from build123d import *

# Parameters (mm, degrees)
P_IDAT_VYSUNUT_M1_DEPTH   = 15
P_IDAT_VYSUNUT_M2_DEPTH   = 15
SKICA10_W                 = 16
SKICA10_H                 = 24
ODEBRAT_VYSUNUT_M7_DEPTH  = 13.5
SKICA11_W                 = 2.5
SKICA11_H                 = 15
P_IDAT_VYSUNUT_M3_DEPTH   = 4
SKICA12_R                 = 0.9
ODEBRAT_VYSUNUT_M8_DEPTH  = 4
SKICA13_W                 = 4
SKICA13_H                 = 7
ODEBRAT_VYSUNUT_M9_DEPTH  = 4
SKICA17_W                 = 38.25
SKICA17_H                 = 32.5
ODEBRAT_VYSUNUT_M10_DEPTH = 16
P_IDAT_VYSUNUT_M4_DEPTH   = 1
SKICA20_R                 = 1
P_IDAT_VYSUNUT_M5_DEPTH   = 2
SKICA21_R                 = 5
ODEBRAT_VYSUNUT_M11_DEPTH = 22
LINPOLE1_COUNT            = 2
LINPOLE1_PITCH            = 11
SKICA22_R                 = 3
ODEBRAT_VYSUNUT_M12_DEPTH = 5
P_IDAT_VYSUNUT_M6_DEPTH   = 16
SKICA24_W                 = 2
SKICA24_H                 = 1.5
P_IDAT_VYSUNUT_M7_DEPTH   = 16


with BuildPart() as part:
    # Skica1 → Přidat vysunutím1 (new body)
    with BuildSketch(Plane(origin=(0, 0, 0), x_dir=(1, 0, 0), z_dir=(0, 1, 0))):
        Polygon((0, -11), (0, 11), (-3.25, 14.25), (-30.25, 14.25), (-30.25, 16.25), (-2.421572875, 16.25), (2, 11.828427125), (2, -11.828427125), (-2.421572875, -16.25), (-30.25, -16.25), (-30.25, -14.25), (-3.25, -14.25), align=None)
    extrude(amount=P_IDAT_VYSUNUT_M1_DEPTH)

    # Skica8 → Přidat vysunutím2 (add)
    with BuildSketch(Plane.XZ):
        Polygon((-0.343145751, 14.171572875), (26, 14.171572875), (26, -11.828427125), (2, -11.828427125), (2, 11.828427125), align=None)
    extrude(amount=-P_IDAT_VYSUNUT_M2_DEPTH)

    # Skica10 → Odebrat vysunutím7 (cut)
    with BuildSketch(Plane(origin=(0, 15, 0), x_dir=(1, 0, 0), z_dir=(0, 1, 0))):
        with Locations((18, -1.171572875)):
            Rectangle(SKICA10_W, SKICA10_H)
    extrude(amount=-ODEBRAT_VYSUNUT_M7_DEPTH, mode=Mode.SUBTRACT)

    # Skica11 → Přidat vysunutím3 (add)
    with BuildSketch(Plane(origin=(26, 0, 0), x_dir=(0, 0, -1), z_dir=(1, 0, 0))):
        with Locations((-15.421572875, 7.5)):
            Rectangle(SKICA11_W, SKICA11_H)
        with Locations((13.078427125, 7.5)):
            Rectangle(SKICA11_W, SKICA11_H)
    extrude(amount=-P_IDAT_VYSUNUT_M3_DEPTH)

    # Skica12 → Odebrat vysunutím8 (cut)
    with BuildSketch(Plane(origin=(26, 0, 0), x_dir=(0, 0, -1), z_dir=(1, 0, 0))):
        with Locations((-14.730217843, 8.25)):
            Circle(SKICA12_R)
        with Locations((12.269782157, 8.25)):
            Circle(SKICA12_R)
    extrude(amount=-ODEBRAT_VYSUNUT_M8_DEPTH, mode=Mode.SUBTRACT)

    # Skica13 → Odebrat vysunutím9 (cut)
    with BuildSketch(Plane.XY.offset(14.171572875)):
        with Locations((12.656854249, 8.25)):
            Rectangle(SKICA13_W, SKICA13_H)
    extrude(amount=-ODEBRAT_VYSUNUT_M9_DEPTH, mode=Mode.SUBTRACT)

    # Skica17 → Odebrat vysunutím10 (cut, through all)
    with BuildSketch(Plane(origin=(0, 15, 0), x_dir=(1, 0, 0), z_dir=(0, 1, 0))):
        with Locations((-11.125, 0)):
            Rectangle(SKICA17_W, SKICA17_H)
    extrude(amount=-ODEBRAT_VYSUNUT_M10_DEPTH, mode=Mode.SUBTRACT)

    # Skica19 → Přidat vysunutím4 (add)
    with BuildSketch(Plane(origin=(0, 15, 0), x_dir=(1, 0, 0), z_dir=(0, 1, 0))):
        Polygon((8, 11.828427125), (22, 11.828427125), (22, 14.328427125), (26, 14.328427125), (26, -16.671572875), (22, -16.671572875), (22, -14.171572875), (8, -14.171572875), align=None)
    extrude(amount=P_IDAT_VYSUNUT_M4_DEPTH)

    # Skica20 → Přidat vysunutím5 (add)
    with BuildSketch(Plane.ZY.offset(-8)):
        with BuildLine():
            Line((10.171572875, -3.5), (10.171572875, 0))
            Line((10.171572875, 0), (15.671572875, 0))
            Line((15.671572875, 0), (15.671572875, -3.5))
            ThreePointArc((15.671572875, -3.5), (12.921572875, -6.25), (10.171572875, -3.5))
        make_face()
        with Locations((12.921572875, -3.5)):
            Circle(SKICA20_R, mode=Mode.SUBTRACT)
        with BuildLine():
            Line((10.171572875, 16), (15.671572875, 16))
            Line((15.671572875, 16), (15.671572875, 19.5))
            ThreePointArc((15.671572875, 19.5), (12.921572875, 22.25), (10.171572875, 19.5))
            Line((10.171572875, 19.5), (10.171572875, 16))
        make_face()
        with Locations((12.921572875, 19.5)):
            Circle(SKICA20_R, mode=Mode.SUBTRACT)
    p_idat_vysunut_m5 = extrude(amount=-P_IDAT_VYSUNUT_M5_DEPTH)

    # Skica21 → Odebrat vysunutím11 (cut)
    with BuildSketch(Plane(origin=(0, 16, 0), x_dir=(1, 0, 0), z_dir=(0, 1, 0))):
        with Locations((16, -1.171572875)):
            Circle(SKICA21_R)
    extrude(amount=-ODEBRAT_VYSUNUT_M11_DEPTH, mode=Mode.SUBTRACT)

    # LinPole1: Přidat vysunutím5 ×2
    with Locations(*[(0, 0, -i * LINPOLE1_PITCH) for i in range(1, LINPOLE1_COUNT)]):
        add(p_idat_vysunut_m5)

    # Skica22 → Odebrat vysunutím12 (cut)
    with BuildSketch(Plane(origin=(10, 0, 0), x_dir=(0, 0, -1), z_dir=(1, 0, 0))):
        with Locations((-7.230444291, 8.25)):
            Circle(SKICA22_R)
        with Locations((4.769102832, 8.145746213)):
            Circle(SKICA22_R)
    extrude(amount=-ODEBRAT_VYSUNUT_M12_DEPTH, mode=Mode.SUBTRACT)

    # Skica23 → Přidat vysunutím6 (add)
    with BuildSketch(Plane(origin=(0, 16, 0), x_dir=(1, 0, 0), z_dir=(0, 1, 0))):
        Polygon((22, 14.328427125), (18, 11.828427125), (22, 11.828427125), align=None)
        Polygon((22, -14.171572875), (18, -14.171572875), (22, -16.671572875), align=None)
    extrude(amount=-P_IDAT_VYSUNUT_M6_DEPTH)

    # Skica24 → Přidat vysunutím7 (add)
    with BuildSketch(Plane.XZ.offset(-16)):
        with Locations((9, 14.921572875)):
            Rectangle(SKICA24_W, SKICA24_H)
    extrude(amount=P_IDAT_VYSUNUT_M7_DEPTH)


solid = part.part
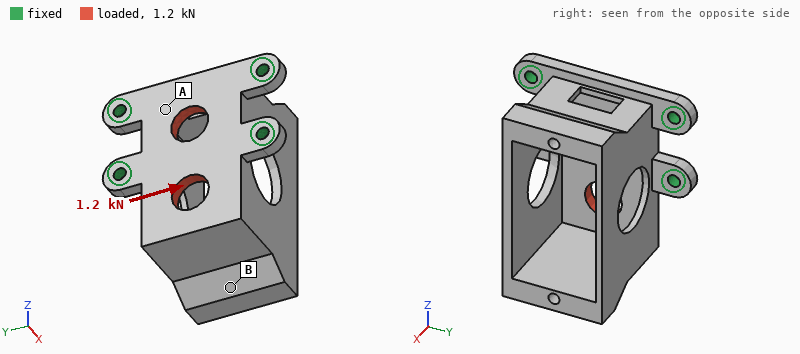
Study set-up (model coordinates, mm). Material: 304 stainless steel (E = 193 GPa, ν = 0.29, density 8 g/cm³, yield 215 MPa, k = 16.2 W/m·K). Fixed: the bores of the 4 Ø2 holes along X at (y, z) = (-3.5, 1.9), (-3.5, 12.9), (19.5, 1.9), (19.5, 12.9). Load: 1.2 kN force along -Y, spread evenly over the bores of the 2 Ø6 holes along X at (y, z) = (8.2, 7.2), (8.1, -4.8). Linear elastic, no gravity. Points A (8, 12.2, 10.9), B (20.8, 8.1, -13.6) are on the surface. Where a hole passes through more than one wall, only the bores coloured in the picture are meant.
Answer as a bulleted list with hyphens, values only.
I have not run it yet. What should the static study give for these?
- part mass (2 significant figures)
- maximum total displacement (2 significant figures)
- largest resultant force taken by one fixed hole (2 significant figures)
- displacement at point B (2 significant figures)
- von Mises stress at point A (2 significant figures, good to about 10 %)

- 22 g
- 5.7 µm
- 460 N
- 5.3 µm
- 15 MPa
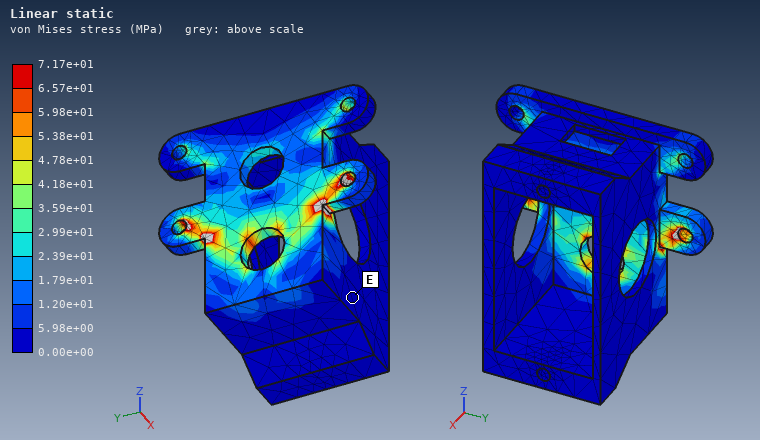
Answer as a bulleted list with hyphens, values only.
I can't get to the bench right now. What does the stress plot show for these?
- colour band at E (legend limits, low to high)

- 0.00e+00 to 5.98e+00 MPa
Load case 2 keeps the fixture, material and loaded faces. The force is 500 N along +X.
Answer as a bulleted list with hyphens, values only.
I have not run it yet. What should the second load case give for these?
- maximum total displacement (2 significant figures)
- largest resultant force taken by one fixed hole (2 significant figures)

- 22 µm
- 240 N
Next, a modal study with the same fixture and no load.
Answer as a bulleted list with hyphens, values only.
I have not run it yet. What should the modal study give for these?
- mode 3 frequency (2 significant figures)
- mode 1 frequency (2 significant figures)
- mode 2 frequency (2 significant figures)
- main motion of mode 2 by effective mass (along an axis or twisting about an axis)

- 9500 Hz
- 5000 Hz
- 5600 Hz
- along Y
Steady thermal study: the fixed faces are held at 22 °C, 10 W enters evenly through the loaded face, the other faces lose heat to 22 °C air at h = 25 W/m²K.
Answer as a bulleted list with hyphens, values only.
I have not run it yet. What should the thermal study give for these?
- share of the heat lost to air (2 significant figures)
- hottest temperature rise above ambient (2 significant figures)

- 36 %
- 89 K
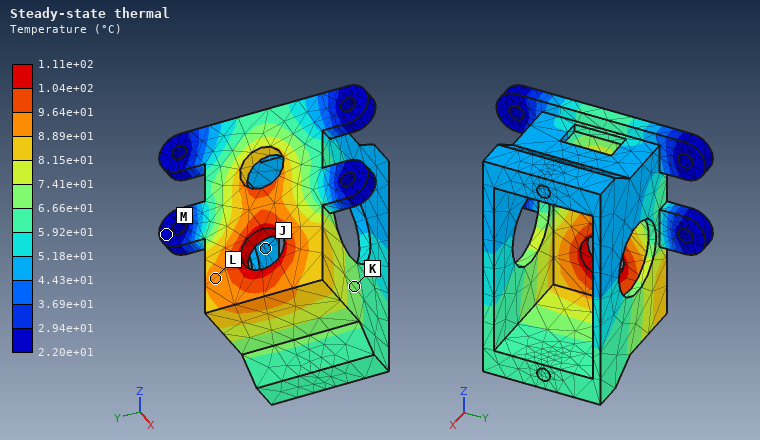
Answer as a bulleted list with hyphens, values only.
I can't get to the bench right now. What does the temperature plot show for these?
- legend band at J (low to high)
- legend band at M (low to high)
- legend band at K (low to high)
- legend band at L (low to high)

- 4.43e+01 to 5.18e+01 °C
- 2.20e+01 to 2.94e+01 °C
- 6.66e+01 to 7.41e+01 °C
- 8.89e+01 to 9.64e+01 °C
